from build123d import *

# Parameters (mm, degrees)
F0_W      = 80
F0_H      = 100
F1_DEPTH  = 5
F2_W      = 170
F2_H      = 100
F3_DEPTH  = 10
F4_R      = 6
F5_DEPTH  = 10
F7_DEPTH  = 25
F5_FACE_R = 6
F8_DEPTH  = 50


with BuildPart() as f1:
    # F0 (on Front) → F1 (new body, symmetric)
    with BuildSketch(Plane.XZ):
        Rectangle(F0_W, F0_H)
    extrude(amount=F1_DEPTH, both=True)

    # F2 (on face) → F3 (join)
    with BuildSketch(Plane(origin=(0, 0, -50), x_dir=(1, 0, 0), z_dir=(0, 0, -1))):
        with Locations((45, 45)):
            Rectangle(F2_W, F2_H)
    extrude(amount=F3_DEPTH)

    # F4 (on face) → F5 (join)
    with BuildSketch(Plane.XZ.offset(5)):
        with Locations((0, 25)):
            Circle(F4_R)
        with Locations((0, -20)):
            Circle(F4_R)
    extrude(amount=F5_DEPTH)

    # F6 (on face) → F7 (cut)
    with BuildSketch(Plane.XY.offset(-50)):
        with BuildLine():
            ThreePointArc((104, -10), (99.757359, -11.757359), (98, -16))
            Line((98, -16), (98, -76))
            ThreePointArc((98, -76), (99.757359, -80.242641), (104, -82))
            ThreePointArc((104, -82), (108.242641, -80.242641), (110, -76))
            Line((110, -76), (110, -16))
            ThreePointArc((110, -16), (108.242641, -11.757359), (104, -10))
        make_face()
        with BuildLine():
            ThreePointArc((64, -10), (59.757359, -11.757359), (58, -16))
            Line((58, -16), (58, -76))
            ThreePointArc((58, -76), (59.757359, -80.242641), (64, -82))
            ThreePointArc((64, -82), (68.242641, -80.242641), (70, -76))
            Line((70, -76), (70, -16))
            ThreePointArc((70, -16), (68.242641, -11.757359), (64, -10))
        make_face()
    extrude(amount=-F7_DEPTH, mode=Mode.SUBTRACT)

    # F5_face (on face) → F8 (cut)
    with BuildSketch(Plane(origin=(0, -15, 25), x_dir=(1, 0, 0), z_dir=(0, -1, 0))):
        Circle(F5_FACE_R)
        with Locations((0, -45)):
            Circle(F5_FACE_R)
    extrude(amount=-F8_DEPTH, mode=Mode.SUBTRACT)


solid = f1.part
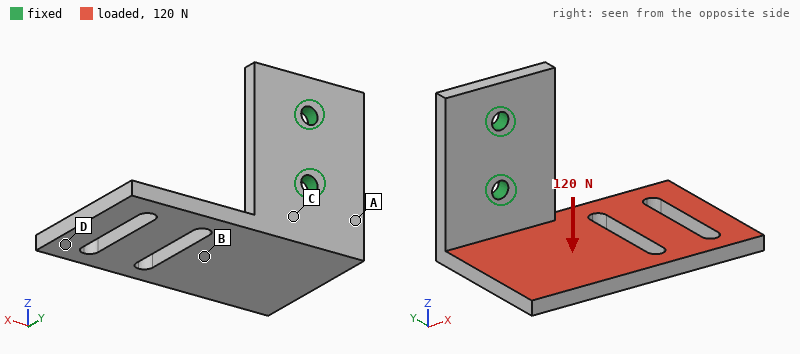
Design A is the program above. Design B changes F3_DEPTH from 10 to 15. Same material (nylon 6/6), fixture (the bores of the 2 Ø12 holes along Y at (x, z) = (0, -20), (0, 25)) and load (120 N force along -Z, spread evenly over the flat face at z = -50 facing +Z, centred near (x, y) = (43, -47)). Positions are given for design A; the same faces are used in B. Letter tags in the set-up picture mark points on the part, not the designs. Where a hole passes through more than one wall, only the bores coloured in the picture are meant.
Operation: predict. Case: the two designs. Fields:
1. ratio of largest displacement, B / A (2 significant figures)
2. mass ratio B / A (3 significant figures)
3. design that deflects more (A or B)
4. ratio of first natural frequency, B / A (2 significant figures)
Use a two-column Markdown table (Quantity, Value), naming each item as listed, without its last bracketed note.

| Quantity | Value |
|---|---|
| ratio of largest displacement, B / A | 0.59 |
| mass ratio B / A | 1.33 |
| design that deflects more | A |
| ratio of first natural frequency, B / A | 0.95 |
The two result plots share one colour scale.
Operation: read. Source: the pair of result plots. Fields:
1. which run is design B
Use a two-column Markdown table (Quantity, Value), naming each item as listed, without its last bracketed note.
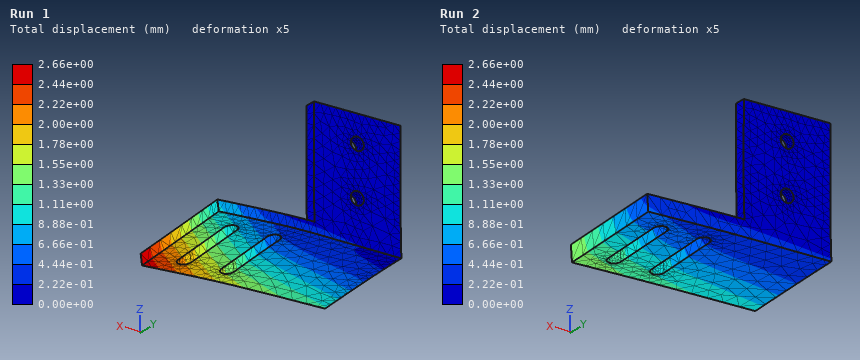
| Quantity | Value |
|---|---|
| which run is design B | Run 2 |
